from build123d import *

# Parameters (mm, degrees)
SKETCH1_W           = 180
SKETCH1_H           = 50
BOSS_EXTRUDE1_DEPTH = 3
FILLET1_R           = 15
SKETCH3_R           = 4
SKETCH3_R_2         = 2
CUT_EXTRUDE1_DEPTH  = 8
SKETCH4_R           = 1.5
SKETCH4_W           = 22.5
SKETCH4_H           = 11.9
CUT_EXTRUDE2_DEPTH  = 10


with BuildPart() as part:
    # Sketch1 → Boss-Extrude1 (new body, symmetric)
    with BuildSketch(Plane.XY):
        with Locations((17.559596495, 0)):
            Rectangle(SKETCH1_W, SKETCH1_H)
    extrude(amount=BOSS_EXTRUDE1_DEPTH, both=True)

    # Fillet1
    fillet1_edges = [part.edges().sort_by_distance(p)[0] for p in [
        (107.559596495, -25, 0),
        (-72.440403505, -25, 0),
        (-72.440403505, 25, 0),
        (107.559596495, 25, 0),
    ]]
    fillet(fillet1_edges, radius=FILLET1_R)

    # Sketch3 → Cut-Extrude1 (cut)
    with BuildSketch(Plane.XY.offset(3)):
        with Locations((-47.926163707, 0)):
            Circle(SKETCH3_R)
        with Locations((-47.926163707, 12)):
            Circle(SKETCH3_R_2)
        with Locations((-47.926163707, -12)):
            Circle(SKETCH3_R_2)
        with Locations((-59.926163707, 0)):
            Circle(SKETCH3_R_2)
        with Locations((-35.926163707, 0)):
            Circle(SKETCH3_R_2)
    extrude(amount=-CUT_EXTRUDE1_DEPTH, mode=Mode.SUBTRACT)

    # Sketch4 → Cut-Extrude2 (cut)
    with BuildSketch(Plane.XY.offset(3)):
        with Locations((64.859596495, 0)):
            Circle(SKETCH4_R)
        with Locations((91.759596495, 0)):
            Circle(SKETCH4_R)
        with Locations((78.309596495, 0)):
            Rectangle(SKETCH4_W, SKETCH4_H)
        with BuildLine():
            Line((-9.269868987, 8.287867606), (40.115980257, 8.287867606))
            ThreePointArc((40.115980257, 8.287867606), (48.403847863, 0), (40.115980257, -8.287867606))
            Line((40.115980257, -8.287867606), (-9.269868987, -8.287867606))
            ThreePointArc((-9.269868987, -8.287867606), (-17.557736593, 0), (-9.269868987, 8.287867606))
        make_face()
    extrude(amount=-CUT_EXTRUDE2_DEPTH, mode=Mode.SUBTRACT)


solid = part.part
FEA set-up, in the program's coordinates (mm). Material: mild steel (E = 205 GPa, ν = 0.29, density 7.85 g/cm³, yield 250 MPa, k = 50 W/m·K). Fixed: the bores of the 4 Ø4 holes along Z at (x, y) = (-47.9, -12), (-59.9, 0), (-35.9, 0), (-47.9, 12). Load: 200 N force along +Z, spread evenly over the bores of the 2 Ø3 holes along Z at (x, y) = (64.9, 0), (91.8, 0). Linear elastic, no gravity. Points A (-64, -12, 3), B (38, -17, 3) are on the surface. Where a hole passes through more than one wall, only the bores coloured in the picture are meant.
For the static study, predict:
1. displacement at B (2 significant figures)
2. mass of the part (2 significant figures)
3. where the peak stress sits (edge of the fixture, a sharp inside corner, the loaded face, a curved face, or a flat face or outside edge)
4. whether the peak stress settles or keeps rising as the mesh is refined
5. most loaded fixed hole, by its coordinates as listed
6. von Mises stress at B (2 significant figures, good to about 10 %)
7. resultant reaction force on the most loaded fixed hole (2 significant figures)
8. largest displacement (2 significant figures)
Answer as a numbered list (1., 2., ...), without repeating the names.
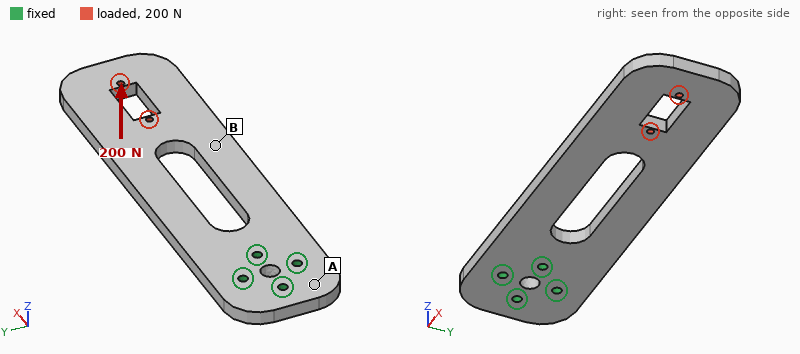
1. 0.35 mm
2. 350 g
3. edge of the fixture
4. keeps rising
5. (-35.9, 0)
6. 41 MPa
7. 1.1 kN
8. 1.0 mm
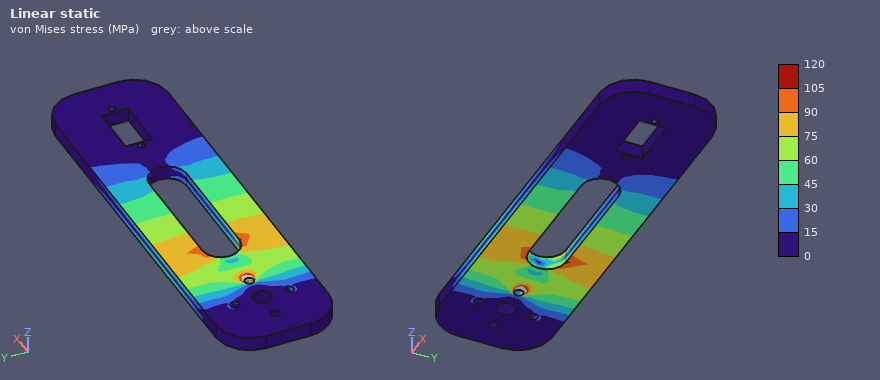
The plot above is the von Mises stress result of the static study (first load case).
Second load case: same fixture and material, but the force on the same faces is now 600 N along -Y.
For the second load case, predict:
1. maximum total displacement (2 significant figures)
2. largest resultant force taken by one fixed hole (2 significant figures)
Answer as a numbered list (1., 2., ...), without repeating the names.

1. 73 µm
2. 1.8 kN
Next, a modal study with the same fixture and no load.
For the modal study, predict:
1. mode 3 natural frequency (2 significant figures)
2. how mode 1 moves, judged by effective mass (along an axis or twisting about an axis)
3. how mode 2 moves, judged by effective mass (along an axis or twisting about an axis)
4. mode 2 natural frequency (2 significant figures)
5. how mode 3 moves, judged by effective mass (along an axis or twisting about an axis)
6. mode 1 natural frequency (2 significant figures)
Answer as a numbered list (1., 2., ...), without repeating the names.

1. 1300 Hz
2. along Z
3. twisting about X
4. 1100 Hz
5. along Y
6. 230 Hz
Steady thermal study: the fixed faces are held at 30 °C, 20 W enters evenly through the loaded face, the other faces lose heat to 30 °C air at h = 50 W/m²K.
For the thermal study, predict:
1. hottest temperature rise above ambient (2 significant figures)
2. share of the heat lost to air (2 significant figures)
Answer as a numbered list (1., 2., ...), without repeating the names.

1. 66 K
2. 89 %
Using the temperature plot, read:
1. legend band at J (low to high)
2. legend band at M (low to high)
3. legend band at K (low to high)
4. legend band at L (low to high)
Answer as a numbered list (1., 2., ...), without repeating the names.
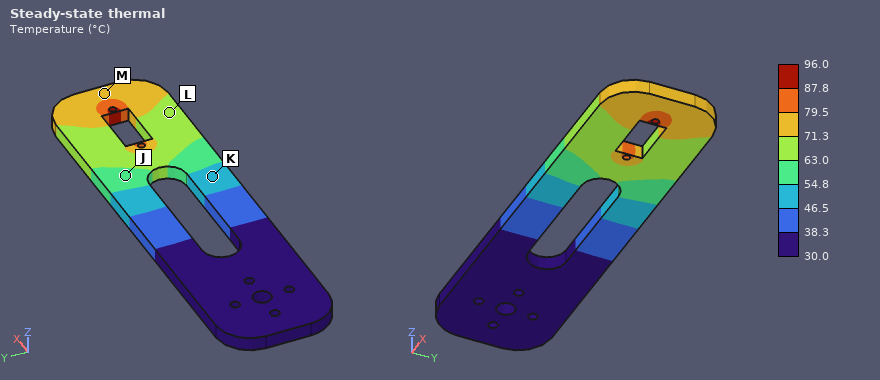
1. 54.8 to 63.0 °C
2. 71.3 to 79.5 °C
3. 46.5 to 54.8 °C
4. 63.0 to 71.3 °C
